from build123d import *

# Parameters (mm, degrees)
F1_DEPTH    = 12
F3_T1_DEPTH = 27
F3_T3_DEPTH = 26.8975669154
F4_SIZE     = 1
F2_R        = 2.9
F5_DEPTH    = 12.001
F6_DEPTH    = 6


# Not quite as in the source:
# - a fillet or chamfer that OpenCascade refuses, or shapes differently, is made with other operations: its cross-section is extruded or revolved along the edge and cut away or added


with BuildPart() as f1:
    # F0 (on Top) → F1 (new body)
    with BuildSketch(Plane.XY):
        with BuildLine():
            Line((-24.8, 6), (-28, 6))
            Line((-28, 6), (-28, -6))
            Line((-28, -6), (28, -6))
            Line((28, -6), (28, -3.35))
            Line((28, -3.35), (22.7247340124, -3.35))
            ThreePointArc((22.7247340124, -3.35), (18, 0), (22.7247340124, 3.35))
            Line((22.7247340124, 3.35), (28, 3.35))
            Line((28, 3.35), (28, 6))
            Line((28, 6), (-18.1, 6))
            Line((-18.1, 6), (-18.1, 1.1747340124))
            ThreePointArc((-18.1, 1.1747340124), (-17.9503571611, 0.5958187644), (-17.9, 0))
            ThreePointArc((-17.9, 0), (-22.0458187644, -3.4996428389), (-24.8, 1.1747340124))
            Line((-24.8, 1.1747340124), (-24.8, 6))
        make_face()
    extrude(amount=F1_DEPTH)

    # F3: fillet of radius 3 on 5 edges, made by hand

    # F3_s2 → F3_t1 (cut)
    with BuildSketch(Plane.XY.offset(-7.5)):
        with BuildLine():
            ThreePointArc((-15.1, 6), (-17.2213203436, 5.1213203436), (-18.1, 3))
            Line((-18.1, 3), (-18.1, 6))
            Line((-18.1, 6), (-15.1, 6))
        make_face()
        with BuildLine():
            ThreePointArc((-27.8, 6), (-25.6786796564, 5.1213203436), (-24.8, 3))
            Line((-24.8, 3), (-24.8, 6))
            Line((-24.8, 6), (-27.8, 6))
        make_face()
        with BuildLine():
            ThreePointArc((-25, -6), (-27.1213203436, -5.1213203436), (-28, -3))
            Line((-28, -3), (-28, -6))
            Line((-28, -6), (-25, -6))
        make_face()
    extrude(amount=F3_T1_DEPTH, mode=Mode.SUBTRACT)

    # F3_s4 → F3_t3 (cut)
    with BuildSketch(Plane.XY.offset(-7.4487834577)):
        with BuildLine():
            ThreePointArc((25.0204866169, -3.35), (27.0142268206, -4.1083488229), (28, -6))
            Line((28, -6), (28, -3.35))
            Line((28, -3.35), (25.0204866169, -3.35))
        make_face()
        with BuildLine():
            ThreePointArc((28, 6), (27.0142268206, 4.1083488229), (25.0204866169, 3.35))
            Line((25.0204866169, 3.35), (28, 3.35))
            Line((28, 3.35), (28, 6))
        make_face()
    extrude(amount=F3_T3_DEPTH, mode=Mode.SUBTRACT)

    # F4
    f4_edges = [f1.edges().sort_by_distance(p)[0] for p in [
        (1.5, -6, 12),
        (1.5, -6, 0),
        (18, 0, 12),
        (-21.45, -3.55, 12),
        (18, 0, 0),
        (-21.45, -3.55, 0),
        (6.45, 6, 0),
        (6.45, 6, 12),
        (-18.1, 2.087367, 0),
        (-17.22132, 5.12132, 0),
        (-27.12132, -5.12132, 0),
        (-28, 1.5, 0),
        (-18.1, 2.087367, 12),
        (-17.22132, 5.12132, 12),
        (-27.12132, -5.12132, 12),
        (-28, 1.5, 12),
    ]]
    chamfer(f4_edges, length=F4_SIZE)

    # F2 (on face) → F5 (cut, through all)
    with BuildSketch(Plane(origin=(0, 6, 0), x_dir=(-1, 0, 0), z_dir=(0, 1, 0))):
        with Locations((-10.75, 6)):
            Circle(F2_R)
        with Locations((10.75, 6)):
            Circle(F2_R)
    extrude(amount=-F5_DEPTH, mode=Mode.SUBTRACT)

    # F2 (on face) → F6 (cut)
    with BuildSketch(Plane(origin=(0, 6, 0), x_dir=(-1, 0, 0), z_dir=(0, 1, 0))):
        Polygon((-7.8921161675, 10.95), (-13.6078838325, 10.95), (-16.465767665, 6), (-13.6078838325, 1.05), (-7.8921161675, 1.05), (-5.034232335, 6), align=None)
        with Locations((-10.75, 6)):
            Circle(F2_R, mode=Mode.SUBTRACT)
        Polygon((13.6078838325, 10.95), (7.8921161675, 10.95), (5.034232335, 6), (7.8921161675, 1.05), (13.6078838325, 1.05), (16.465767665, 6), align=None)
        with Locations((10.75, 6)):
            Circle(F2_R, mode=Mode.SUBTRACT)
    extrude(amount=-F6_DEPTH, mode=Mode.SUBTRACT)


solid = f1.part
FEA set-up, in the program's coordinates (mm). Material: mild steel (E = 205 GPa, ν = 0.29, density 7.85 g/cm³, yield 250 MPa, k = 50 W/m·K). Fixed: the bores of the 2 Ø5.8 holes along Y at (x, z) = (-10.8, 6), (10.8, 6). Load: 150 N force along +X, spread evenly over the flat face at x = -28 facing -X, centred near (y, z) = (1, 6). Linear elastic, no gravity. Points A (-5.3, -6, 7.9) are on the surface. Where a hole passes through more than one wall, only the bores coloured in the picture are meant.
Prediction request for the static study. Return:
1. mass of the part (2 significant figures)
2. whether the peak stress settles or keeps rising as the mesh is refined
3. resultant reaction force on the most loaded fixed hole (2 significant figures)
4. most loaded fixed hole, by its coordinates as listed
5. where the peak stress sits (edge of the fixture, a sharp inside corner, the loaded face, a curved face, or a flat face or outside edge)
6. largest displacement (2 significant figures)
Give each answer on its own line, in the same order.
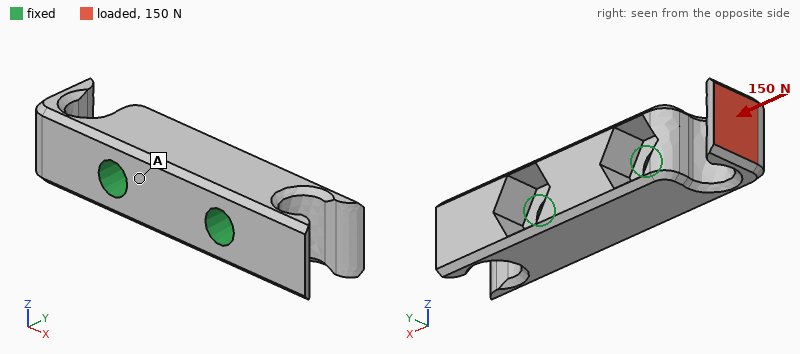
39 g
keeps rising
140 N
(-10.8, 6)
a sharp inside corner
24 µm
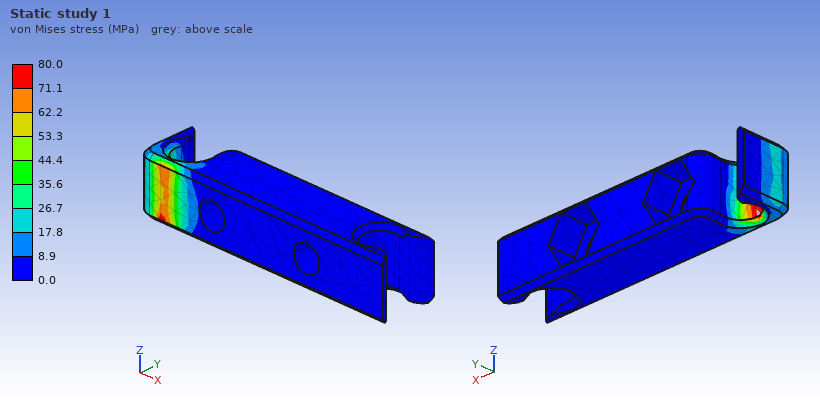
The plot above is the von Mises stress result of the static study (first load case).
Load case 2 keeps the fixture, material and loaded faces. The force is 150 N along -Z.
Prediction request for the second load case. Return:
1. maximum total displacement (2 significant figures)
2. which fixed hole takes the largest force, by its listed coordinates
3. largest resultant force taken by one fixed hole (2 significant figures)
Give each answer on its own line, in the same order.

12 µm
(-10.8, 6)
180 N
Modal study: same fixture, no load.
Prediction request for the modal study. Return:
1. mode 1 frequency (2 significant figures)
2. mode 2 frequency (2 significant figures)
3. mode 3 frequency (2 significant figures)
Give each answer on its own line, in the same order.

8000 Hz
13 kHz
18 kHz
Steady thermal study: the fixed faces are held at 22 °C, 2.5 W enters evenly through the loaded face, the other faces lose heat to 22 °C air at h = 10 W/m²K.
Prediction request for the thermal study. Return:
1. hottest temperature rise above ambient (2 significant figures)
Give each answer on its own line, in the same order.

23 K
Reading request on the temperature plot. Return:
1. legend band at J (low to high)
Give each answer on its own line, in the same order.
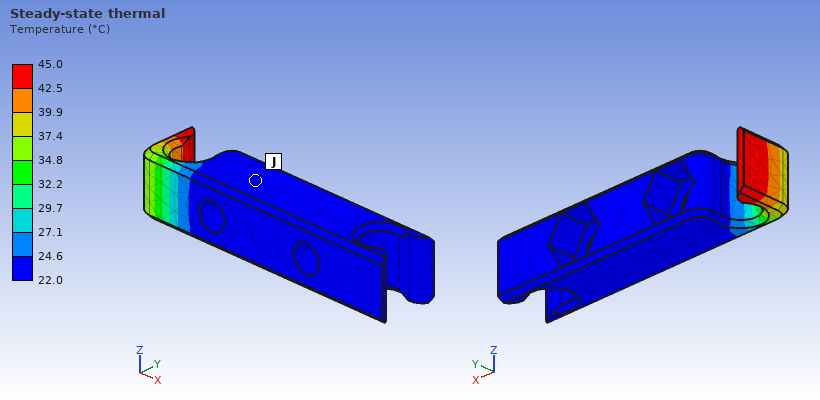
22.0 to 24.6 °C
